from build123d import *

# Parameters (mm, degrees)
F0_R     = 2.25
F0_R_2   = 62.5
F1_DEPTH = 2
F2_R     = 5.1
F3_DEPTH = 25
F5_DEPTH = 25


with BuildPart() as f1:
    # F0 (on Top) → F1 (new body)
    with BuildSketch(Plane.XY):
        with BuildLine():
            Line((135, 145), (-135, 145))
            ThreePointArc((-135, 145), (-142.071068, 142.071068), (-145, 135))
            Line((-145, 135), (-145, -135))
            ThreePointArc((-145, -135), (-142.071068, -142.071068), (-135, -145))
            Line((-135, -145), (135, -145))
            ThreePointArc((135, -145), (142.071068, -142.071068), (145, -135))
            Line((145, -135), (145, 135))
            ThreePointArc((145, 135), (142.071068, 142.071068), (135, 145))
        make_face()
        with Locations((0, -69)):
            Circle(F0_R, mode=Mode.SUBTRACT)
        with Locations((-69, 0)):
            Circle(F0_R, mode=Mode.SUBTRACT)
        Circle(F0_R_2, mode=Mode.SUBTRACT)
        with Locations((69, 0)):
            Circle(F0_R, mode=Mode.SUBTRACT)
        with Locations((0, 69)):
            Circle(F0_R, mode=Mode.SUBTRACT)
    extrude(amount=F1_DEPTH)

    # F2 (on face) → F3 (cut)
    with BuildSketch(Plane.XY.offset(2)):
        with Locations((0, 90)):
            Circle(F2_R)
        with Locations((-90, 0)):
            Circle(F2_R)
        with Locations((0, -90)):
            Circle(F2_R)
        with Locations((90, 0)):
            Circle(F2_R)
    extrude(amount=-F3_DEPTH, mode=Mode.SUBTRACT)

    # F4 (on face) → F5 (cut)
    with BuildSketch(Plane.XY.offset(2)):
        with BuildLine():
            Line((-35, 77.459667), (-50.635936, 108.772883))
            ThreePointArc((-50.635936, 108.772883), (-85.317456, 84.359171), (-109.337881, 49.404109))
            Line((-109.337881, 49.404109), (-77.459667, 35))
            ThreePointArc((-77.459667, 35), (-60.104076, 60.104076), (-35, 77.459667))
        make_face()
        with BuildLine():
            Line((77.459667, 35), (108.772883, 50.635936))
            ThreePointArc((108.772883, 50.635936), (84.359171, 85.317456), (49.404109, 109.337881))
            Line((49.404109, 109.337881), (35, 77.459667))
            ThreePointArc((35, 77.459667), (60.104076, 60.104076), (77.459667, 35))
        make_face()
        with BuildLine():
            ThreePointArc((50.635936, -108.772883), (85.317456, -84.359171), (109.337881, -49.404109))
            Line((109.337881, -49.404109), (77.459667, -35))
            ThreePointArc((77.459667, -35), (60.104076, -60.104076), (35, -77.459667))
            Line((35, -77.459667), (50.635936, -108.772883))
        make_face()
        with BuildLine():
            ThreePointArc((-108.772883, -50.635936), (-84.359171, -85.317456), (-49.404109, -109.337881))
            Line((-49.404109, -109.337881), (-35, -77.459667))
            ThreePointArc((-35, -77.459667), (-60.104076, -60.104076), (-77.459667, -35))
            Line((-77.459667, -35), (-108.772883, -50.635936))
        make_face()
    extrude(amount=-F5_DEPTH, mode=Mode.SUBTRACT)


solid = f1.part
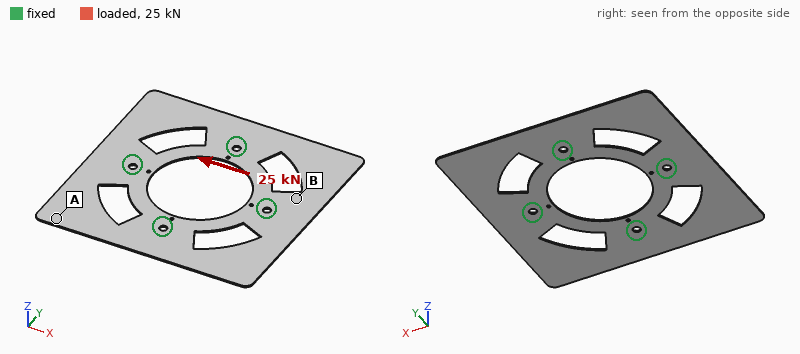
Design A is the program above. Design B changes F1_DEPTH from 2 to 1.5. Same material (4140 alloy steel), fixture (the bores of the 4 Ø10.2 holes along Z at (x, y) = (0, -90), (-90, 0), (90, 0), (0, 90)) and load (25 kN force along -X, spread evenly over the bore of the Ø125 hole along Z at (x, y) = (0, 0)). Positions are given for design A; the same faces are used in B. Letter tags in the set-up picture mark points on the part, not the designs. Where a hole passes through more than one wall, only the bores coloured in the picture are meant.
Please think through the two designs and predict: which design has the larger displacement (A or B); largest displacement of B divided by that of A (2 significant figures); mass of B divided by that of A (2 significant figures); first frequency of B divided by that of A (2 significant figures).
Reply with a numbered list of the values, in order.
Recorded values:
1. B
2. 1.3
3. 0.75
4. 0.75
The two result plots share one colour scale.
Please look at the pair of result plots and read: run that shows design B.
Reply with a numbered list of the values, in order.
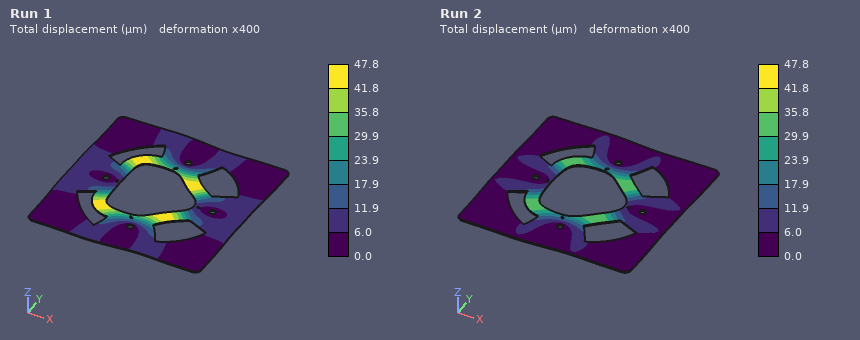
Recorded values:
1. Run 1
